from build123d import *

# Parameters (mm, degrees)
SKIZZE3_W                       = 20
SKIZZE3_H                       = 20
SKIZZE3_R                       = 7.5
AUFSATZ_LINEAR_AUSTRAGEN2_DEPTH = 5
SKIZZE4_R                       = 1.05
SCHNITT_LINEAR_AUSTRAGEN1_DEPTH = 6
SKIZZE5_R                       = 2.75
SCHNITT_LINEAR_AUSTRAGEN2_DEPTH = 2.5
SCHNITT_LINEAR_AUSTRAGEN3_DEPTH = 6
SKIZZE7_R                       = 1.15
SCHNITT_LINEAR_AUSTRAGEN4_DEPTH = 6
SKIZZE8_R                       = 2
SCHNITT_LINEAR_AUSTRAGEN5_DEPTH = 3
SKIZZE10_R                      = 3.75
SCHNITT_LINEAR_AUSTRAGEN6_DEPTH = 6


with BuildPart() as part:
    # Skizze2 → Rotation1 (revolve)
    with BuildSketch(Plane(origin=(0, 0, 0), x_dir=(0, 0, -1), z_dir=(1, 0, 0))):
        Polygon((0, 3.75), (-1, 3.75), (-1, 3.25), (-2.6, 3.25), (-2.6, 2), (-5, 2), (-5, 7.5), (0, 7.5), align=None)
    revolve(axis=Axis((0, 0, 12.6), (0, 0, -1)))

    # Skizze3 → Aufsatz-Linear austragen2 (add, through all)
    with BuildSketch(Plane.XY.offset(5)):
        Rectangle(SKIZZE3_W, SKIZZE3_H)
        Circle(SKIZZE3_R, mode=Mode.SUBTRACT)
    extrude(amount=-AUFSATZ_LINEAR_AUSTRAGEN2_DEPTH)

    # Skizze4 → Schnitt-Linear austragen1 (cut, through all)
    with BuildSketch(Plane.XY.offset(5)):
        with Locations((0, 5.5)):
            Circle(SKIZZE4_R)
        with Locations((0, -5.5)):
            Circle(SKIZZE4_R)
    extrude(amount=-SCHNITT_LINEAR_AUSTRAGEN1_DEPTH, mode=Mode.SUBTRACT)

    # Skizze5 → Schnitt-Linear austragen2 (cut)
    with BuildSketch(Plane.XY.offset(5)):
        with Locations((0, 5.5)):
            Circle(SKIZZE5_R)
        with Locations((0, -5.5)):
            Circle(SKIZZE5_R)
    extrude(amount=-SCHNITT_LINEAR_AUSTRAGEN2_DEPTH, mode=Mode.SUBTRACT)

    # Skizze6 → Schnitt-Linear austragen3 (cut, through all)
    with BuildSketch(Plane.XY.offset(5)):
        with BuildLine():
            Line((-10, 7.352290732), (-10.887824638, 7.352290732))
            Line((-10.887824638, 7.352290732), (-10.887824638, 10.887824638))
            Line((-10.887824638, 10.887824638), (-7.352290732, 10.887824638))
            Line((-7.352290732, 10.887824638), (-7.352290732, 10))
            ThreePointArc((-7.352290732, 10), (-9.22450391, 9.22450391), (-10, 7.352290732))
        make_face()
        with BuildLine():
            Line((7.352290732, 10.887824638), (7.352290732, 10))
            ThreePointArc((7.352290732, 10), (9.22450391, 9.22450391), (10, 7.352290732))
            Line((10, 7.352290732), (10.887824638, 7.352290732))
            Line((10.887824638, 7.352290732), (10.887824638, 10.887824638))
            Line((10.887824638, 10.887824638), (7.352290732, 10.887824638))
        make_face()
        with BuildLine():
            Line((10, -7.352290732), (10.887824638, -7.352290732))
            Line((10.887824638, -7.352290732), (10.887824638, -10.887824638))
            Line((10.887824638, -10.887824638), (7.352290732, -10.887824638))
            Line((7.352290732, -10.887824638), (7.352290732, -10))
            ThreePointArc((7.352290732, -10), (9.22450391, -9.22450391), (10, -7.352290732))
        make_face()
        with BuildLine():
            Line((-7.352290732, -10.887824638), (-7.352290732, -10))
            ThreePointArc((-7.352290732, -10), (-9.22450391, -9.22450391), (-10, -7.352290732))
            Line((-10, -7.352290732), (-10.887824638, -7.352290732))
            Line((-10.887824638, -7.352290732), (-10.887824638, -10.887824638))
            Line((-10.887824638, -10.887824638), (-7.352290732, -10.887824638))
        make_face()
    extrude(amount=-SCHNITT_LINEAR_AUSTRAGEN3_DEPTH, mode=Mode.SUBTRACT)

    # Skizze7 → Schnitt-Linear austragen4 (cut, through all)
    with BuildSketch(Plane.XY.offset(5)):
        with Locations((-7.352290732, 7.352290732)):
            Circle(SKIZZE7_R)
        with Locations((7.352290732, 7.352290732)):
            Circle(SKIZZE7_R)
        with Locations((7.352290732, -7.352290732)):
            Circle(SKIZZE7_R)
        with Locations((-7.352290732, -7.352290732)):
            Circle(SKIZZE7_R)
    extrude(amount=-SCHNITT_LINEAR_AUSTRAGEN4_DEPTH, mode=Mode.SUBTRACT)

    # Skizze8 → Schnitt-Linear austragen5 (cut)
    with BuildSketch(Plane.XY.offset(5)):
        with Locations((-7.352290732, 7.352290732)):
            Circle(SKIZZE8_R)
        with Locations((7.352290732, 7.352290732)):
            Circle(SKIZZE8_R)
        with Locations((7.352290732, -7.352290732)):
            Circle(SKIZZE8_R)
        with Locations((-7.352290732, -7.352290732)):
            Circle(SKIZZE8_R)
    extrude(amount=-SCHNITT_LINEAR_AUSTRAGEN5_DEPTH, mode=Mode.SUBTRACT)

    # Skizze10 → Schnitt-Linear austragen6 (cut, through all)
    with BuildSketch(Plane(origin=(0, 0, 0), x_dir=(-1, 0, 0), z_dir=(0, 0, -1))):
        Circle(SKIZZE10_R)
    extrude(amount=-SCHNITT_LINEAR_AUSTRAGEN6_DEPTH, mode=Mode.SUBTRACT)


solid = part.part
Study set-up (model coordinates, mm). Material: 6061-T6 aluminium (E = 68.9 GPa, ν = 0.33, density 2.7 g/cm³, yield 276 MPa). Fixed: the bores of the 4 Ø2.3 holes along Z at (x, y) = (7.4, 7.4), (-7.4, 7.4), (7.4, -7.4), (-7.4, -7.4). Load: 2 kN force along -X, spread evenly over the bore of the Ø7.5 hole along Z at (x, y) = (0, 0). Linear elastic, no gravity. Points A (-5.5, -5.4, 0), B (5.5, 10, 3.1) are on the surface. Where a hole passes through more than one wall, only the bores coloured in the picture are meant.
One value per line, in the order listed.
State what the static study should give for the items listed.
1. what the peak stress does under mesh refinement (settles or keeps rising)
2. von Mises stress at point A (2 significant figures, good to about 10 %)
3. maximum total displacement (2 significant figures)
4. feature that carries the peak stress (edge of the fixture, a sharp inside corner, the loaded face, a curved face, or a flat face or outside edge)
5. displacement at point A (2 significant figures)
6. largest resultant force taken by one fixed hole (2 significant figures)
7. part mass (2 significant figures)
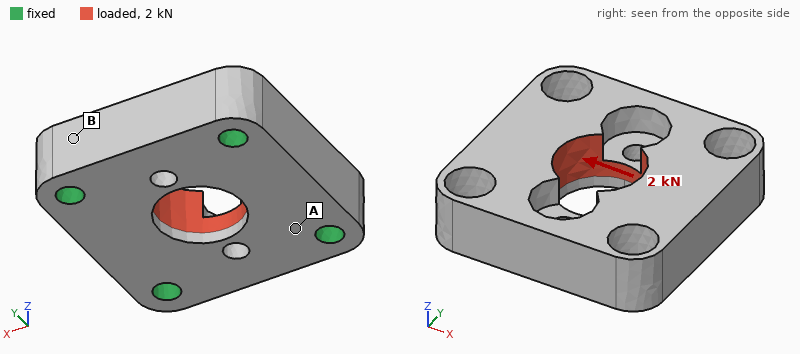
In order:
keeps rising
31 MPa
8.3 µm
edge of the fixture
1.6 µm
530 N
3.9 g
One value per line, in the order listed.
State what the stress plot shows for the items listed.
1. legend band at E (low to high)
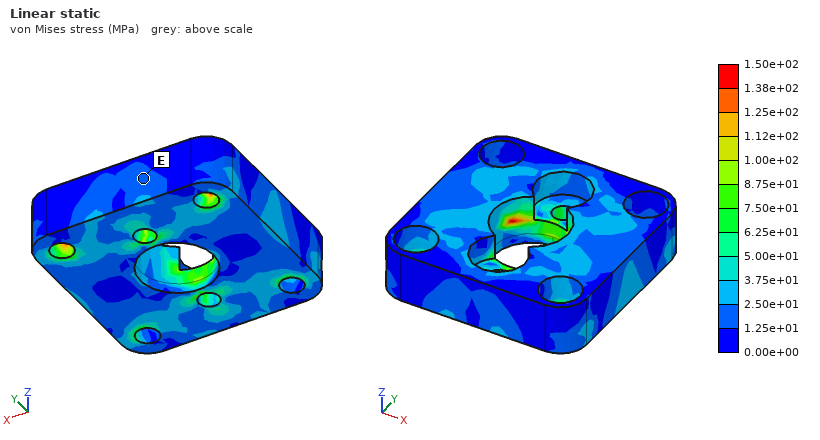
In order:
1.25e+01 to 2.50e+01 MPa
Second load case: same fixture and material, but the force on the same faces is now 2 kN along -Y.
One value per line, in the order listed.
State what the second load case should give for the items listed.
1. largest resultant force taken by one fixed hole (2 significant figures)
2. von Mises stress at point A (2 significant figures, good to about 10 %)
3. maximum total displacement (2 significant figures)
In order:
540 N
33 MPa
6.2 µm
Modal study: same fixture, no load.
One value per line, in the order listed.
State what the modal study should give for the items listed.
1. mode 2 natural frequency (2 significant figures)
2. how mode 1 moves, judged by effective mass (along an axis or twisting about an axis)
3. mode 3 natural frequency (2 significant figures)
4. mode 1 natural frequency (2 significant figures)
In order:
59 kHz
along Z
61 kHz
43 kHz
